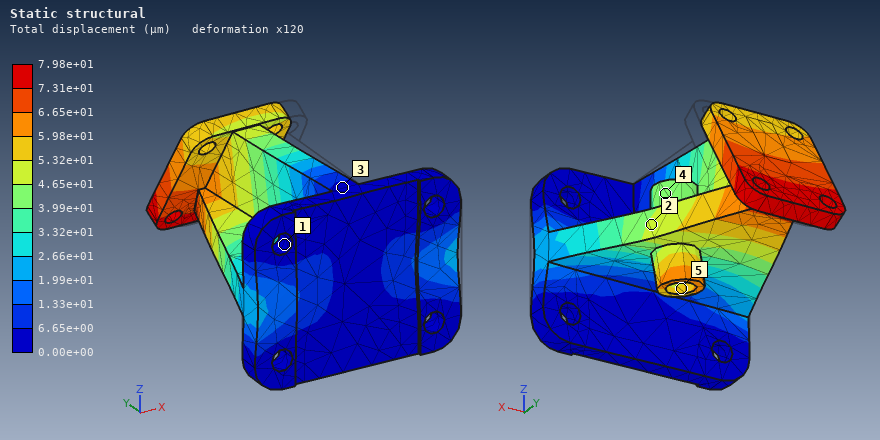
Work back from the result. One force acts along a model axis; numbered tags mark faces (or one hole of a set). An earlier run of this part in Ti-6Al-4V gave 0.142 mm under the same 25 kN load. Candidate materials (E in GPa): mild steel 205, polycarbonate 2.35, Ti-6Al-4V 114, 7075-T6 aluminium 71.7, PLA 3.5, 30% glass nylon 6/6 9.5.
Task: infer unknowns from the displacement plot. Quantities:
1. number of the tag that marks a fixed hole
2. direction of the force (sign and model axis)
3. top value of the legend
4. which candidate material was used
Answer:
1
-X
7.98e+01 µm
mild steel
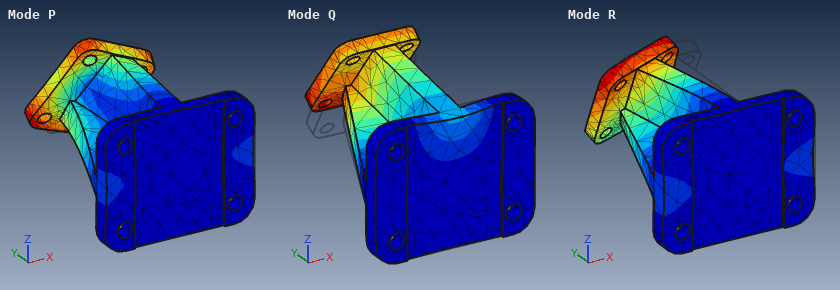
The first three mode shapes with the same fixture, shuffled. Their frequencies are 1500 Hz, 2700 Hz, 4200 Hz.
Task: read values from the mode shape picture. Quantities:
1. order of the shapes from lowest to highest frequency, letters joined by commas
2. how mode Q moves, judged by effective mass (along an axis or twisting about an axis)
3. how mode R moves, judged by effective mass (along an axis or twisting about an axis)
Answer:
Q, R, P
along Z
along X
